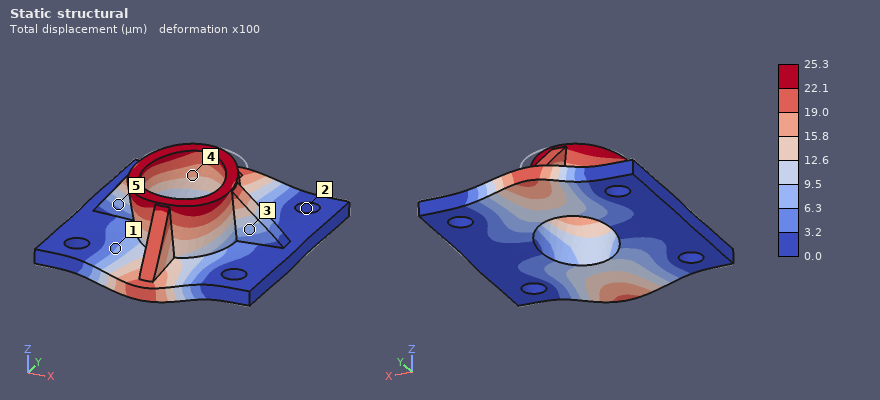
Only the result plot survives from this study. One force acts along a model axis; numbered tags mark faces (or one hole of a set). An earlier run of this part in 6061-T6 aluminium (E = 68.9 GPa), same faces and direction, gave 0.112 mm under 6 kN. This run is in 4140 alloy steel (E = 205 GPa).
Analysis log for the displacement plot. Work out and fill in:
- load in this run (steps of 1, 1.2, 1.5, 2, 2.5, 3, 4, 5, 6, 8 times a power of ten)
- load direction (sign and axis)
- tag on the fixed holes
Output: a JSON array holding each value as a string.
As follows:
["4 kN", "-Y", "2"]
